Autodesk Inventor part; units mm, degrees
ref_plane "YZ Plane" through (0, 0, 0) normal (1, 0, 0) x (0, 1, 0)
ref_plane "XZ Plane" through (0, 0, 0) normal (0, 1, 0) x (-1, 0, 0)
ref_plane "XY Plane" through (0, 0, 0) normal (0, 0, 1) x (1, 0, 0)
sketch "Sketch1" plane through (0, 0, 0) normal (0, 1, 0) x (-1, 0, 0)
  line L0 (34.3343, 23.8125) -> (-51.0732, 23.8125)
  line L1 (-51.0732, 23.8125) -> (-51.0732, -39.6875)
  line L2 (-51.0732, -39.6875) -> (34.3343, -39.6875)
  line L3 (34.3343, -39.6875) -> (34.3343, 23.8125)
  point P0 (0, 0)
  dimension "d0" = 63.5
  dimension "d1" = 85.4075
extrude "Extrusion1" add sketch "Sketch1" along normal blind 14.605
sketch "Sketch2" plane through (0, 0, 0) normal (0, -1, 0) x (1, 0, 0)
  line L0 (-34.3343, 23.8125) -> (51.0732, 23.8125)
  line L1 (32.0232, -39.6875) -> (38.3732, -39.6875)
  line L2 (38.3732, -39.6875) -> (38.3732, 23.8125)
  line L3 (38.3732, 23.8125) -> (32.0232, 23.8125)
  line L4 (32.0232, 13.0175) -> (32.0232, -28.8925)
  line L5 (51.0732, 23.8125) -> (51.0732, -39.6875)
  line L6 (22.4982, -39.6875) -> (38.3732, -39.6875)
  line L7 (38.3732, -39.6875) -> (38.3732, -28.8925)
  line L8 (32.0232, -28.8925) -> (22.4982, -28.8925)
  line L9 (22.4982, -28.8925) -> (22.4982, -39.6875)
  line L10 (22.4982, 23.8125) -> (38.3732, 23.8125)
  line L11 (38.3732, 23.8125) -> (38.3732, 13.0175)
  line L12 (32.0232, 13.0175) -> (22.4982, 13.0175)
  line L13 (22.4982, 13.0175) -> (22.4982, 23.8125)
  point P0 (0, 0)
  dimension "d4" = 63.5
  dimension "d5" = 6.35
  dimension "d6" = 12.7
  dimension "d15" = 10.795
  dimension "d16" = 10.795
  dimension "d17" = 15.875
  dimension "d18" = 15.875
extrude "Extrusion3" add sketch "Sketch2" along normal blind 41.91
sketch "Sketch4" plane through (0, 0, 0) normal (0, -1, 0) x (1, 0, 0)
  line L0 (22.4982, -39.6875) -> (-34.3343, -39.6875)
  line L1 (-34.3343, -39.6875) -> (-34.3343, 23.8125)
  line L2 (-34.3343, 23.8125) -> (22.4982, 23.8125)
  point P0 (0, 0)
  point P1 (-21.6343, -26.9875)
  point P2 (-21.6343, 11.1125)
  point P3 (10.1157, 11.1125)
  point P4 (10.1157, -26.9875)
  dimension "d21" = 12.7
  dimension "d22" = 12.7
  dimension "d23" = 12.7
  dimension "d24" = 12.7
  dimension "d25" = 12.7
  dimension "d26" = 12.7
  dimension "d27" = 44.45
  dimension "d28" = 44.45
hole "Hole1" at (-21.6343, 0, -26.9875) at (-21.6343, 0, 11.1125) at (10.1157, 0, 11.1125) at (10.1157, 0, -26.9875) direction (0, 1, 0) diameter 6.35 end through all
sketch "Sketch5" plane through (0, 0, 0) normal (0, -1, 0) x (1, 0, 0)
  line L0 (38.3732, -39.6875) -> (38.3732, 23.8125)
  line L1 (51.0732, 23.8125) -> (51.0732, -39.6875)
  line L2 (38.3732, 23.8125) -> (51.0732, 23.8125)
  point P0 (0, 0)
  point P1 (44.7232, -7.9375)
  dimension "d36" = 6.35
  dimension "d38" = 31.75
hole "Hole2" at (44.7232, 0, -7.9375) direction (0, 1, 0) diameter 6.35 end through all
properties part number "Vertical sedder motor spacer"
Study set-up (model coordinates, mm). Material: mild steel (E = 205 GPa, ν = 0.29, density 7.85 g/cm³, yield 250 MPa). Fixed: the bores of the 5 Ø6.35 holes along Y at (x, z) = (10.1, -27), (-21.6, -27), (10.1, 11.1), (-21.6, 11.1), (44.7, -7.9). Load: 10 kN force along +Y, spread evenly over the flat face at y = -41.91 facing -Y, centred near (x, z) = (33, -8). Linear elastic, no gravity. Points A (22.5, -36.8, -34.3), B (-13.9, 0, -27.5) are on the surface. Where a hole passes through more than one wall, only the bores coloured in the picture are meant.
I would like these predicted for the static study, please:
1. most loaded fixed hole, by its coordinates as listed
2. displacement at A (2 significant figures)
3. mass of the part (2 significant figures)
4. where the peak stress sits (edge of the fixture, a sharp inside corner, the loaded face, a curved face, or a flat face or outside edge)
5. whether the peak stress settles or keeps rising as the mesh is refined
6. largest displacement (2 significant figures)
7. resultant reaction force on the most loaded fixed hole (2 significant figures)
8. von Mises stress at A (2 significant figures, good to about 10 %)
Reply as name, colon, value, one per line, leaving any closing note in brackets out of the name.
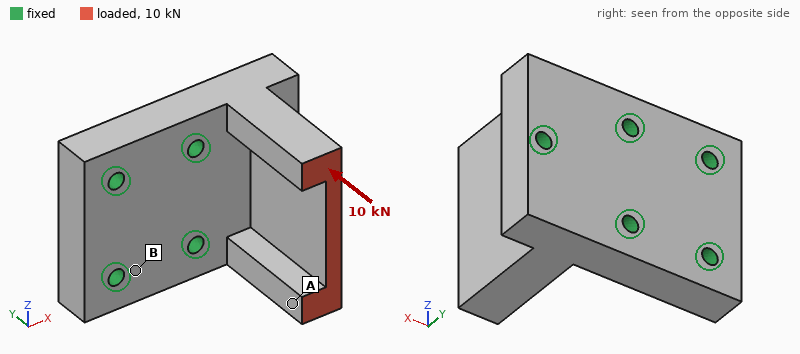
most loaded fixed hole, by its coordinates as listed: (44.7, -7.9)
displacement at A: 6.6 µm
mass of the part: 800 g
where the peak stress sits: edge of the fixture
whether the peak stress settles or keeps rising as the mesh is refined: keeps rising
largest displacement: 7.2 µm
resultant reaction force on the most loaded fixed hole: 5.6 kN
von Mises stress at A: 17 MPa
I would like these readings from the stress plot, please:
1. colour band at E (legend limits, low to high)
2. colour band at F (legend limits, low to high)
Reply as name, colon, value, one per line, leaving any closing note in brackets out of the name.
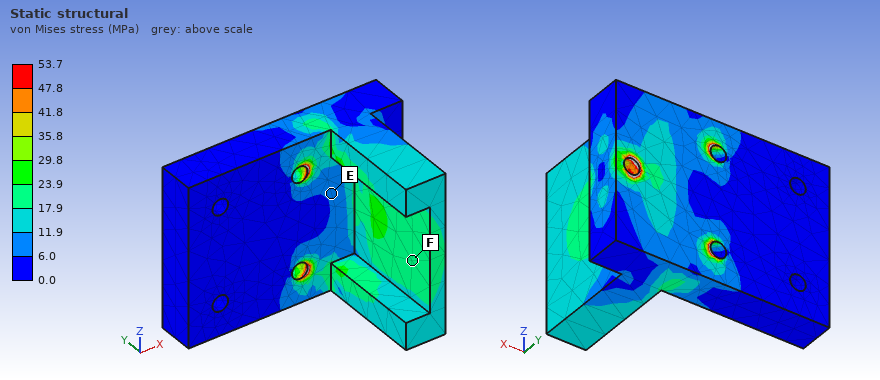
colour band at E: 6.0 to 11.9 MPa
colour band at F: 17.9 to 23.9 MPa
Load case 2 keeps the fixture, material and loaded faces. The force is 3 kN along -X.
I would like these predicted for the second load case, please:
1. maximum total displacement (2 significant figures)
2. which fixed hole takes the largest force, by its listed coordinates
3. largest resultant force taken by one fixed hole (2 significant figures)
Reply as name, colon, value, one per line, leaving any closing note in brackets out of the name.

maximum total displacement: 69 µm
which fixed hole takes the largest force, by its listed coordinates: (44.7, -7.9)
largest resultant force taken by one fixed hole: 4.8 kN
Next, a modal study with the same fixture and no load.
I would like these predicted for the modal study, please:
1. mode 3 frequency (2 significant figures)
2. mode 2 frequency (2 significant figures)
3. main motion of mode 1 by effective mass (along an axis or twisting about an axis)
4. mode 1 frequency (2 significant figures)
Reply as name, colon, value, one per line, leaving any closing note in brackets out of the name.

mode 3 frequency: 7900 Hz
mode 2 frequency: 5300 Hz
main motion of mode 1 by effective mass: along X
mode 1 frequency: 4700 Hz
